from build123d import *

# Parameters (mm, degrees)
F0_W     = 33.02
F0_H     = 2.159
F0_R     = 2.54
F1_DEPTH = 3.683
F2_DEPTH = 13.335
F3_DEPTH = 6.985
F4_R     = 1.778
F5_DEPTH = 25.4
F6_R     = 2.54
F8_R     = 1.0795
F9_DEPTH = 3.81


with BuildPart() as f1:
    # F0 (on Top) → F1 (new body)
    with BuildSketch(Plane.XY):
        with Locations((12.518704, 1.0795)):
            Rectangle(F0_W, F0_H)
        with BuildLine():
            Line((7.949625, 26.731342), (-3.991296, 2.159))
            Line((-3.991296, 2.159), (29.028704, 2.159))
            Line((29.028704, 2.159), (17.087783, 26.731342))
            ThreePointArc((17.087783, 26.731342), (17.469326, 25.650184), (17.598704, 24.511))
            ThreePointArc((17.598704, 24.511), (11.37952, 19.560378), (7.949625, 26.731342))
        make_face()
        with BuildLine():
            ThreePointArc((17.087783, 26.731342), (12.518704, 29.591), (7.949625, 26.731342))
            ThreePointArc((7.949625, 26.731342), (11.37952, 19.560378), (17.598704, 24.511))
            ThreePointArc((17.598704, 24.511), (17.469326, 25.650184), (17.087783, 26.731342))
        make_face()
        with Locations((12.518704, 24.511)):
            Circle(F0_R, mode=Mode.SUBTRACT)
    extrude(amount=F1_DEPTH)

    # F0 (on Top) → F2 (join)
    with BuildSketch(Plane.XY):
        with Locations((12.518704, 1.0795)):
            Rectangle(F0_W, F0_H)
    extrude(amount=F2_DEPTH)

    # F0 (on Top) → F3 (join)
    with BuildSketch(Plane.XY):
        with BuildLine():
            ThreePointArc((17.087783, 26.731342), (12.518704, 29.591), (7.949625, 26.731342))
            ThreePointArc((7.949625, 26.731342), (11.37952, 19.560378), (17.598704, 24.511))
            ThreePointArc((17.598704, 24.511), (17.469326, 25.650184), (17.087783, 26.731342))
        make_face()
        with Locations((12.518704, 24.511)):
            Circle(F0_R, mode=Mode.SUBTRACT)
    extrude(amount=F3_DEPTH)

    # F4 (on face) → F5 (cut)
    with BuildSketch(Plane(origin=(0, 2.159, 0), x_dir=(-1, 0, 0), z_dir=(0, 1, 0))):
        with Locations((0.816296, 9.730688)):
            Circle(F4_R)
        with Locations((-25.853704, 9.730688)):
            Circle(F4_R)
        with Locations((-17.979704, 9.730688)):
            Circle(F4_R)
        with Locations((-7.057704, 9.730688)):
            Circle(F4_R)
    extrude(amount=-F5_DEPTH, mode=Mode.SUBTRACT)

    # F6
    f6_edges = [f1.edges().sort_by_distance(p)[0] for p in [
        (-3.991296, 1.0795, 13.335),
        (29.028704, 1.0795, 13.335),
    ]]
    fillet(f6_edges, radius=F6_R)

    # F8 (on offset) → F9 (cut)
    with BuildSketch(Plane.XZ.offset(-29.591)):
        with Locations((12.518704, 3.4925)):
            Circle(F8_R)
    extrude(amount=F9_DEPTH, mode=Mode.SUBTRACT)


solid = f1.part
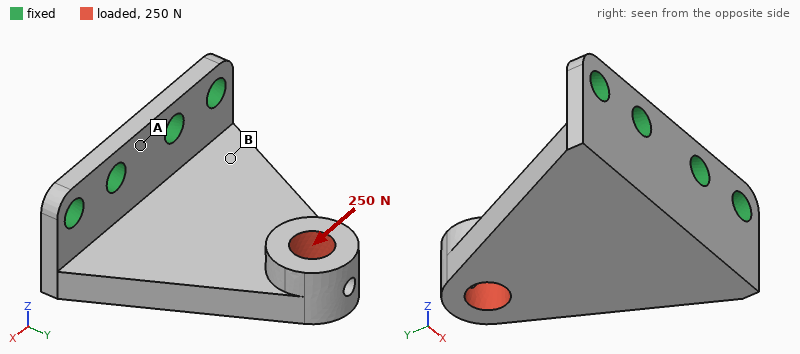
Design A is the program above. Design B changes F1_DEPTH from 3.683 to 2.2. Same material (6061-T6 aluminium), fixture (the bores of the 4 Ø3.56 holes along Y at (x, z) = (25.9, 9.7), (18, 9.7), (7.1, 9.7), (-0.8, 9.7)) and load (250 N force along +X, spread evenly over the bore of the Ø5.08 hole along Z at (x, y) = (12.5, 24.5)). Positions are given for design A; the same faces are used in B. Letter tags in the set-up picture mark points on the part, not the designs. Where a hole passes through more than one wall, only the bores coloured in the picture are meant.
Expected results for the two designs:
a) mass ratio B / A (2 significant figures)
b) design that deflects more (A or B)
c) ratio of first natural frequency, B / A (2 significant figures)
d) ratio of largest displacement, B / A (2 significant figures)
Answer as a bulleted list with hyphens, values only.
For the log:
- 0.77
- B
- 0.80
- 2.5
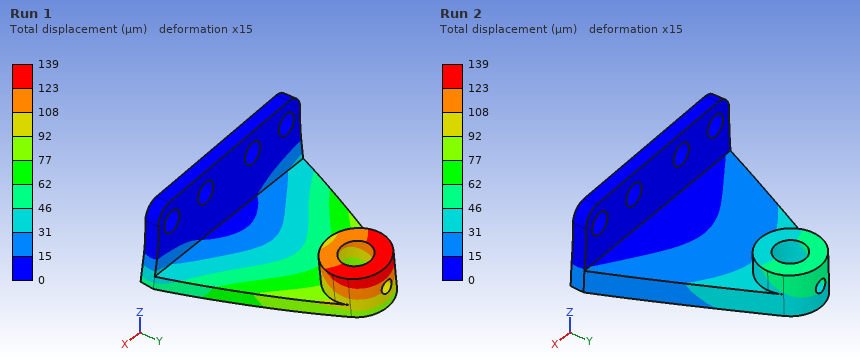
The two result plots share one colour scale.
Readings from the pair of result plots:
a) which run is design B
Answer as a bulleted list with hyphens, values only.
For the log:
- Run 1
